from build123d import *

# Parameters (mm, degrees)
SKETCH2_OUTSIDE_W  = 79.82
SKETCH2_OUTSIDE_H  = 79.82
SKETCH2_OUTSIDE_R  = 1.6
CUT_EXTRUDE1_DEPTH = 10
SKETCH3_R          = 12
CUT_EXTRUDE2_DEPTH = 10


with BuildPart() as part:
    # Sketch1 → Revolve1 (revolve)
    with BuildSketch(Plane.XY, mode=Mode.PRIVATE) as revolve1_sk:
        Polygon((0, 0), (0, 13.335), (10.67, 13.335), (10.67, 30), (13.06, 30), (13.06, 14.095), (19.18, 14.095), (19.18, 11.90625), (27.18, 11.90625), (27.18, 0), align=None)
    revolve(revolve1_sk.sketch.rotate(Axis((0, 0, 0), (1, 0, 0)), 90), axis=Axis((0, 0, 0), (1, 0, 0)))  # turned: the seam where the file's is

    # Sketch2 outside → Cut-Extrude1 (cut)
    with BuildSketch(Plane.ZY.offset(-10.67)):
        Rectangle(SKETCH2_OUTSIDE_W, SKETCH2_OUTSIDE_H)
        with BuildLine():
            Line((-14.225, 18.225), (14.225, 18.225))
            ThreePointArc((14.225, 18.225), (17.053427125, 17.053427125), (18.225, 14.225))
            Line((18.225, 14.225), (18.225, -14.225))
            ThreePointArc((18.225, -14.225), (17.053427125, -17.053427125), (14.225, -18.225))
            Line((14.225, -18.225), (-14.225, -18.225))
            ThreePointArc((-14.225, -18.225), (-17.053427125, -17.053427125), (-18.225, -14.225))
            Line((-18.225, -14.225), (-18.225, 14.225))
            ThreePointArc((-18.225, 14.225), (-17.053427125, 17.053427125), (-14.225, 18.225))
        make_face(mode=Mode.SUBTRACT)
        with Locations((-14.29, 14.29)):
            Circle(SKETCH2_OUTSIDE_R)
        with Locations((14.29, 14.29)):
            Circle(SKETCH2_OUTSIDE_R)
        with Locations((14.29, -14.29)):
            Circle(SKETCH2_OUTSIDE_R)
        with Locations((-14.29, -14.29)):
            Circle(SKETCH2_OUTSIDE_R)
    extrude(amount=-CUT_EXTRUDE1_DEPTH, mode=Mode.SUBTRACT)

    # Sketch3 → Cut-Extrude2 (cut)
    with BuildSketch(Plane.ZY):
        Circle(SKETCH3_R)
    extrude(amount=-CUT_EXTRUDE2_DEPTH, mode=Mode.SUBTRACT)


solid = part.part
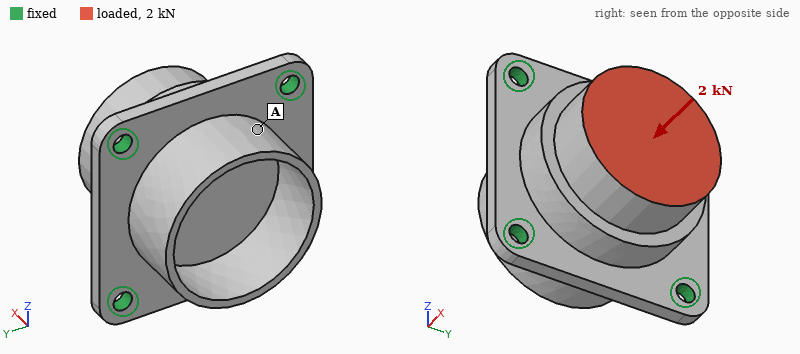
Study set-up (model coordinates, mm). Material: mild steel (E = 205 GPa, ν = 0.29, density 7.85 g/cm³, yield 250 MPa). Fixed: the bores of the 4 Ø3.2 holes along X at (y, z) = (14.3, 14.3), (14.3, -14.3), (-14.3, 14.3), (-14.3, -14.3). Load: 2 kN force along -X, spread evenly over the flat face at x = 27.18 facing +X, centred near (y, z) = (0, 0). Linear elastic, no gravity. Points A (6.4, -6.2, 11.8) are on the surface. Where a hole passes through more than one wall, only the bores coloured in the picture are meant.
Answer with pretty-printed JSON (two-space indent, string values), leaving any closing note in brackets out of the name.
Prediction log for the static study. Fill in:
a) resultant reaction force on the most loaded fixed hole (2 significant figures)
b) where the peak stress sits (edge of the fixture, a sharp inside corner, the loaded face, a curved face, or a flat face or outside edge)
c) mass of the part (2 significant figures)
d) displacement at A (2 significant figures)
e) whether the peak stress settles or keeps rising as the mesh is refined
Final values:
{
  "resultant reaction force on the most loaded fixed hole": "520 N",
  "where the peak stress sits": "edge of the fixture",
  "mass of the part": "93 g",
  "displacement at A": "6.4 µm",
  "whether the peak stress settles or keeps rising as the mesh is refined": "keeps rising"
}
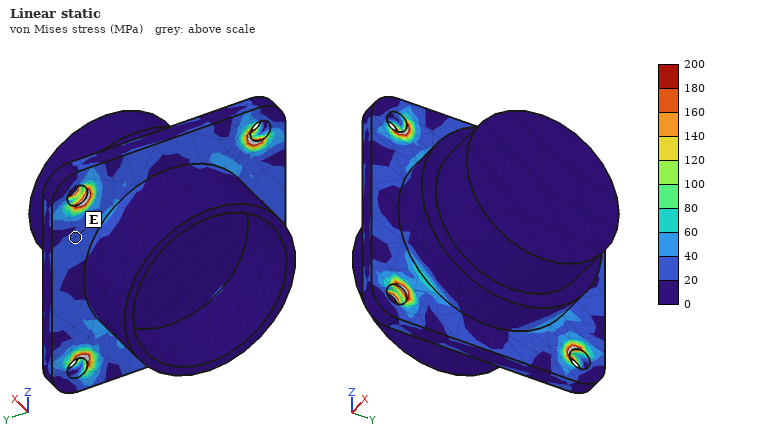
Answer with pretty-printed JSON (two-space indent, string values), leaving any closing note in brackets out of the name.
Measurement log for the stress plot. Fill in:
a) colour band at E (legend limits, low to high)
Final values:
{
  "colour band at E": "20 to 40 MPa"
}
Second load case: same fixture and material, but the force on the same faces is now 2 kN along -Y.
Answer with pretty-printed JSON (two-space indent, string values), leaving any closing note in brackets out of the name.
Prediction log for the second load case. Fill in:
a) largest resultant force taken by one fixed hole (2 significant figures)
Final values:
{
  "largest resultant force taken by one fixed hole": "830 N"
}
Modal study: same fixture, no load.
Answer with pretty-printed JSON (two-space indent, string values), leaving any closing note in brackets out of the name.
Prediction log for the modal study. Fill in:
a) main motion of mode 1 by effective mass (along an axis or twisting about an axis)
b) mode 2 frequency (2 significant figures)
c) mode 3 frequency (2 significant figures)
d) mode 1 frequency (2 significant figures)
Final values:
{
  "main motion of mode 1 by effective mass": "along X",
  "mode 2 frequency": "11 kHz",
  "mode 3 frequency": "11 kHz",
  "mode 1 frequency": "9400 Hz"
}
